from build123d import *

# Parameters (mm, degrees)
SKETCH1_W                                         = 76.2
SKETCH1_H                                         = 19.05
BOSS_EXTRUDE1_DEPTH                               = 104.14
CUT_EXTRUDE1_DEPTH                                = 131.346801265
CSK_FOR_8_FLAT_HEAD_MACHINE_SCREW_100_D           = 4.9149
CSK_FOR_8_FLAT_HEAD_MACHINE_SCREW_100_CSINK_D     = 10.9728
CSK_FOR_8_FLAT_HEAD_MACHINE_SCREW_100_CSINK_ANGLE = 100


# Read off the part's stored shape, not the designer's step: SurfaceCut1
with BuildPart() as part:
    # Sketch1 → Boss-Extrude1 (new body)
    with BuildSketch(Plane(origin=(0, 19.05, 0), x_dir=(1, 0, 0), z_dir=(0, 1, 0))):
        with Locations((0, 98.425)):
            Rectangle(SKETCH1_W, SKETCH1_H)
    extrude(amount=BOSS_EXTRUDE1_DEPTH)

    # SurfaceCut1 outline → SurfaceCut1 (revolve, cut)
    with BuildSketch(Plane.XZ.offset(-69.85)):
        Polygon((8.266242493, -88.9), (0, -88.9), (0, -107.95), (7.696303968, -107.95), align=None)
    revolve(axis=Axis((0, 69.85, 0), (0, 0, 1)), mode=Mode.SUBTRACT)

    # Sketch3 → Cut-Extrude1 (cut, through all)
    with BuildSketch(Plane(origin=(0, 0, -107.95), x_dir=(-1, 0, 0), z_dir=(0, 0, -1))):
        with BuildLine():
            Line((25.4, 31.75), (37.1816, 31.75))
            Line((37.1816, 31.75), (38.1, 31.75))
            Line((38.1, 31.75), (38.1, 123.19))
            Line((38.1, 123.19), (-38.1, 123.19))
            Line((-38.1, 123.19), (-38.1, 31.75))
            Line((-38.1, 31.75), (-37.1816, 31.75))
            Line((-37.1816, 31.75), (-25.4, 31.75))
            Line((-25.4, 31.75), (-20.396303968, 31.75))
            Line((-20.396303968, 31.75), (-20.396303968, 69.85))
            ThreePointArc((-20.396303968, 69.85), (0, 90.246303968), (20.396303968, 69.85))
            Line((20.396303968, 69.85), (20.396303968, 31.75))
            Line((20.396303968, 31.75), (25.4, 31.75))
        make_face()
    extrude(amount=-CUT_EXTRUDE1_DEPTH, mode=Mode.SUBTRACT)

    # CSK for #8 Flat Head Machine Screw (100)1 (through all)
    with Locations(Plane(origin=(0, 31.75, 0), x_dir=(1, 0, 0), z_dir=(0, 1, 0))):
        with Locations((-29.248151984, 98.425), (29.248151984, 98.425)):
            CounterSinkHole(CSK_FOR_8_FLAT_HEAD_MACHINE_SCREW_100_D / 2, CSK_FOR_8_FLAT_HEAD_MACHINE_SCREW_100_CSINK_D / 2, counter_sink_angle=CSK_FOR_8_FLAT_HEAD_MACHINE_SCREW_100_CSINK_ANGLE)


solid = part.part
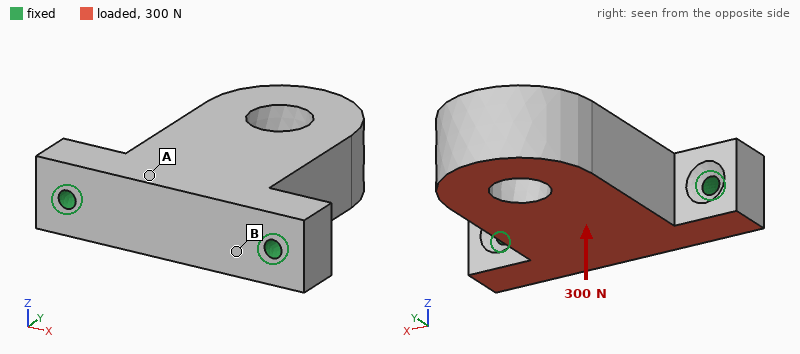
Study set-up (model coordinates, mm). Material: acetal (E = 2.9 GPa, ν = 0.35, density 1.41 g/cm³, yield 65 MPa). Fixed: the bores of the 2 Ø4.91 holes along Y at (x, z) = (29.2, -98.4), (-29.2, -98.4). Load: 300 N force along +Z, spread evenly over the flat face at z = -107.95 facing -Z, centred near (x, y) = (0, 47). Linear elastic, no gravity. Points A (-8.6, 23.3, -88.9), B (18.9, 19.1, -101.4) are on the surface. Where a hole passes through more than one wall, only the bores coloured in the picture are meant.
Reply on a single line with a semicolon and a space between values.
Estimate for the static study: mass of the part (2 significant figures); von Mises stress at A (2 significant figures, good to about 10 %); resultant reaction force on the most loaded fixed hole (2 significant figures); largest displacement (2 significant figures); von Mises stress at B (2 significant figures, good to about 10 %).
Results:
79 g; 1.5 MPa; 150 N; 0.52 mm; 3.6 MPa
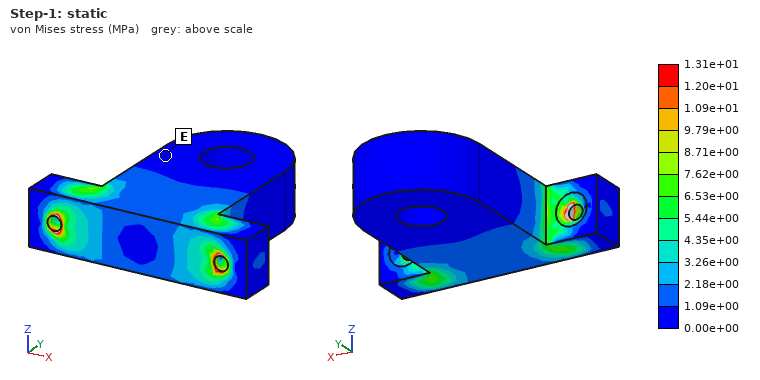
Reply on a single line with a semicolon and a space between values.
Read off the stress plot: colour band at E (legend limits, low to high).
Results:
0.00e+00 to 1.09e+00 MPa
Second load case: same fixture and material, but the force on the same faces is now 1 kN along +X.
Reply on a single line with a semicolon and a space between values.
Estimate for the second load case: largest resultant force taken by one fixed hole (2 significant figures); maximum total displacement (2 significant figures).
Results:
680 N; 0.21 mm
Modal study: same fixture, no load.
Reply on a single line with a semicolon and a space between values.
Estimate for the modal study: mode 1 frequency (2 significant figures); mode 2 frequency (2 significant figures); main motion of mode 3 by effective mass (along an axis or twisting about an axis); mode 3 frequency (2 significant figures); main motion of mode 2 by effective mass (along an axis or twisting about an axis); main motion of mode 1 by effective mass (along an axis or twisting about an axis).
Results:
540 Hz; 1600 Hz; along Y; 2600 Hz; along X; along Z
